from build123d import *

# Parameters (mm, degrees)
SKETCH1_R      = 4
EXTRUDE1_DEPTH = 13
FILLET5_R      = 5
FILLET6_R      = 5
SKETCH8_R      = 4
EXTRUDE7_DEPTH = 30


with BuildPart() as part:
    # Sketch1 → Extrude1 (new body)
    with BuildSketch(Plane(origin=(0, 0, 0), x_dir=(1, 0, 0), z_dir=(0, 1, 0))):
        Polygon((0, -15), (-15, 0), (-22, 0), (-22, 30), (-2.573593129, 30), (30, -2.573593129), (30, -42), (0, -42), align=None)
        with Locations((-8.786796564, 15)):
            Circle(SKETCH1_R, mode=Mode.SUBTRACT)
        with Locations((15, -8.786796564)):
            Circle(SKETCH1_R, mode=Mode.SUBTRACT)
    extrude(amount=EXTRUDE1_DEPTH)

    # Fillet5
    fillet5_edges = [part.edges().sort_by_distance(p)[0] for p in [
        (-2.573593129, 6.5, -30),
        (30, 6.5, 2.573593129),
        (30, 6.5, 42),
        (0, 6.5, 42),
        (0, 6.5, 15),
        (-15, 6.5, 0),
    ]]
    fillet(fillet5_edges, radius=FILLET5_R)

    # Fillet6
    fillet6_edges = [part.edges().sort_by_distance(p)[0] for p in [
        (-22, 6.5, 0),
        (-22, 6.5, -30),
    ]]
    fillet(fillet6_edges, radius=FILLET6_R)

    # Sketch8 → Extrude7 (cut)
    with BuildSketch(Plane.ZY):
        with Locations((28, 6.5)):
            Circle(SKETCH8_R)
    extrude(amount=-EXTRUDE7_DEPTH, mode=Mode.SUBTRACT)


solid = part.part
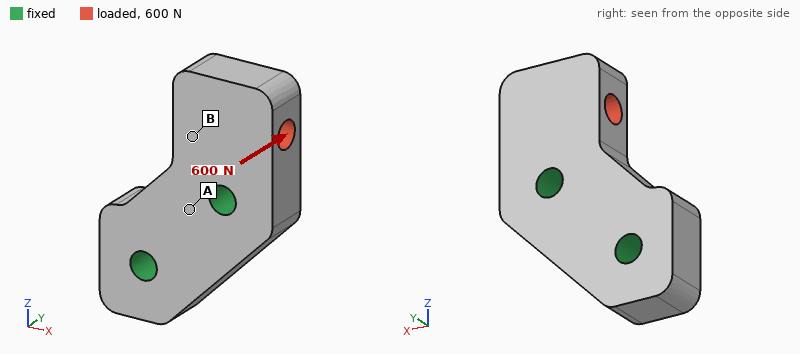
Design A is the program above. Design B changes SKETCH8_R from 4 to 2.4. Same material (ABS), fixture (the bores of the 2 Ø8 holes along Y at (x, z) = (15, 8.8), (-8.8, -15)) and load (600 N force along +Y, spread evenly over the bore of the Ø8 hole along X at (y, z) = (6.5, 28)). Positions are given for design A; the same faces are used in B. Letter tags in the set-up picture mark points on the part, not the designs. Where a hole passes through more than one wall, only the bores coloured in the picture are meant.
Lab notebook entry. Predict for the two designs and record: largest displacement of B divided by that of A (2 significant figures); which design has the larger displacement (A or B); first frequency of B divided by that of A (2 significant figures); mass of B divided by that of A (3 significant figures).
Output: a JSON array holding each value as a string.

["0.84", "A", "1.1", "1.03"]
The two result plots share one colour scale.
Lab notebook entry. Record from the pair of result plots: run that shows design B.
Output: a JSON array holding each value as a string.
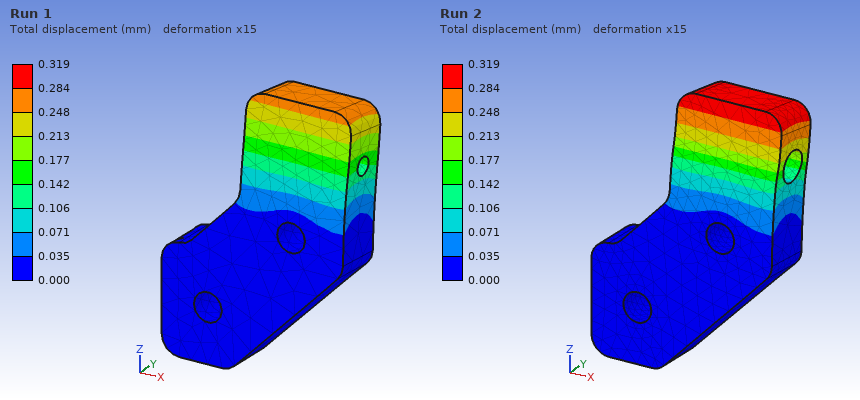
["Run 1"]
